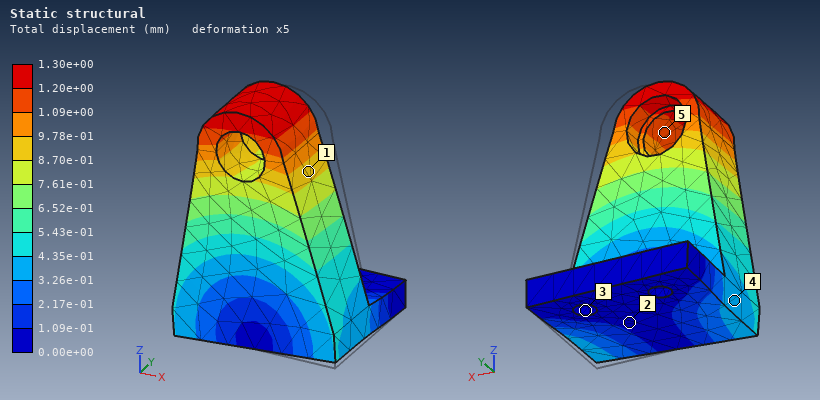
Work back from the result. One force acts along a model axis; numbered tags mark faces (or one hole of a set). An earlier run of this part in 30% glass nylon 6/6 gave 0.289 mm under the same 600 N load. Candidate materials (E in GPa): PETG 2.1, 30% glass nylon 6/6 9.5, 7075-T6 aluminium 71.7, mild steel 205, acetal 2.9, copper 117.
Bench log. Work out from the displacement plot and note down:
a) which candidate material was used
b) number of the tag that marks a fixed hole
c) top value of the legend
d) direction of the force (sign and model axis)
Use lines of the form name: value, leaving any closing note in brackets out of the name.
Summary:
which candidate material was used: PETG
number of the tag that marks a fixed hole: 3
top value of the legend: 1.30e+00 mm
direction of the force: -X
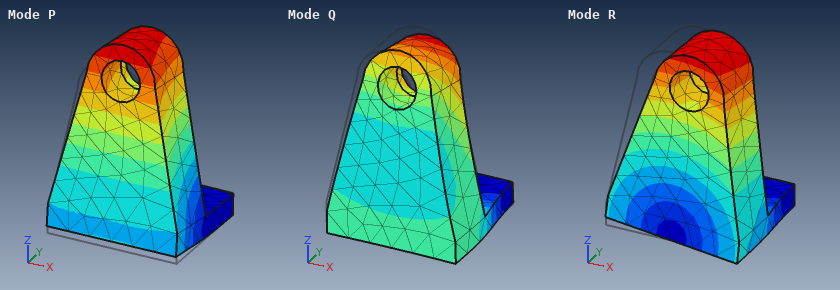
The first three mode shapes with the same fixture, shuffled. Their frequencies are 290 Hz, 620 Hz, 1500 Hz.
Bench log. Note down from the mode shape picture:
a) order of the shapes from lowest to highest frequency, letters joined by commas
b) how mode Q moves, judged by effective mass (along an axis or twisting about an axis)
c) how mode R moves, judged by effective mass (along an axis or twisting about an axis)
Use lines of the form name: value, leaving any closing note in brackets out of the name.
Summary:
order of the shapes from lowest to highest frequency, letters joined by commas: P, R, Q
how mode Q moves, judged by effective mass: along Z
how mode R moves, judged by effective mass: along X
